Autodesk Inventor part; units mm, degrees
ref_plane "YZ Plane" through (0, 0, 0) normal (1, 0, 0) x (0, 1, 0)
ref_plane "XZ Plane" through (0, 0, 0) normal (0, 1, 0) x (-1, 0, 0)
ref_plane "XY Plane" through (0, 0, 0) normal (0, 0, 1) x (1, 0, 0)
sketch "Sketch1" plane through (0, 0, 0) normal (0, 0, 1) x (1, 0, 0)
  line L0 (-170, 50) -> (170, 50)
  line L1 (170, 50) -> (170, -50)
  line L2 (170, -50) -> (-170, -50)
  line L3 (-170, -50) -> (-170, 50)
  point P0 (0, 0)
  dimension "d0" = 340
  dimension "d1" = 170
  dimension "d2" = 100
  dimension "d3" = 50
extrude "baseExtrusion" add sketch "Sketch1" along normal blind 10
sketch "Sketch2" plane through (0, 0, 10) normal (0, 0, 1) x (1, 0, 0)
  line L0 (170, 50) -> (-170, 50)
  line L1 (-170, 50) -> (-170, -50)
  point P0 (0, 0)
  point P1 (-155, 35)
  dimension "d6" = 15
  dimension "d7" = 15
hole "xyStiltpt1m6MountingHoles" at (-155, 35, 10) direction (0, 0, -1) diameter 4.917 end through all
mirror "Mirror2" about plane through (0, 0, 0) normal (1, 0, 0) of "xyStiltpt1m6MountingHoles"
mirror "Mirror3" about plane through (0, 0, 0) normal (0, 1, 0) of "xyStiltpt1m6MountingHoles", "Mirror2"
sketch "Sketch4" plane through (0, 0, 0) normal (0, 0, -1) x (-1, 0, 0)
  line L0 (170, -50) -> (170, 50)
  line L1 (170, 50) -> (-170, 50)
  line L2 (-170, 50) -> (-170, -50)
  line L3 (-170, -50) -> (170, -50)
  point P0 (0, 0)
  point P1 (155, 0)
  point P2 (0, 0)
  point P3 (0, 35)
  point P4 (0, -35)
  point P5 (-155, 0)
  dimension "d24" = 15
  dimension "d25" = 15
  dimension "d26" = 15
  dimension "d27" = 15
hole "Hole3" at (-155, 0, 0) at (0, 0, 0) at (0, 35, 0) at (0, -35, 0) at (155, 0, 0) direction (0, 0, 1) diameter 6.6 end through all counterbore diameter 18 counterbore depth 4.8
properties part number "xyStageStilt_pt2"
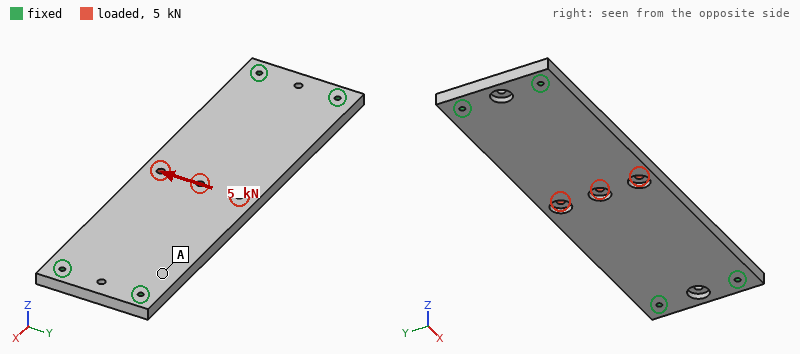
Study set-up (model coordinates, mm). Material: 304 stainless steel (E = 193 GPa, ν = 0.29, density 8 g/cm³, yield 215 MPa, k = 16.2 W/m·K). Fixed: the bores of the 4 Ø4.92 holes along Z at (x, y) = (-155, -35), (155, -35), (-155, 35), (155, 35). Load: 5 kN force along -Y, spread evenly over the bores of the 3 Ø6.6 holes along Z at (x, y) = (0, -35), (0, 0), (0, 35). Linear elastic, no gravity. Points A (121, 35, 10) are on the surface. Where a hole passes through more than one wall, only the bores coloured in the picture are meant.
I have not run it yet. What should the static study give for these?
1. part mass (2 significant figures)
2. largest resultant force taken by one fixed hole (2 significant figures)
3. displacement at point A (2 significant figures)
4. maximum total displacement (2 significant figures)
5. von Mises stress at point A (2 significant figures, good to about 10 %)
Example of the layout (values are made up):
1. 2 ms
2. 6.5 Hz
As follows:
1. 2.7 kg
2. 2.9 kN
3. 3.5 µm
4. 21 µm
5. 6.7 MPa
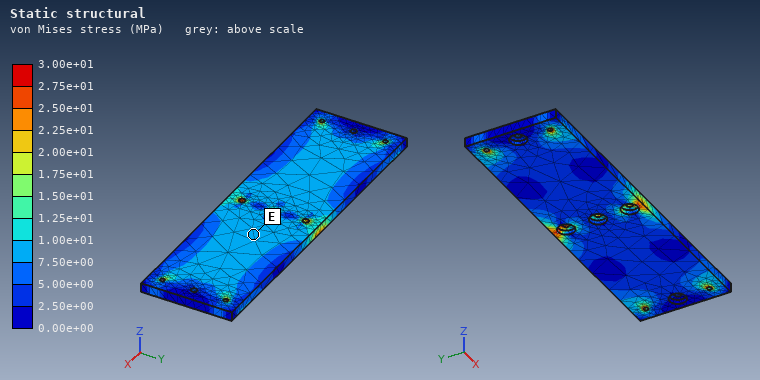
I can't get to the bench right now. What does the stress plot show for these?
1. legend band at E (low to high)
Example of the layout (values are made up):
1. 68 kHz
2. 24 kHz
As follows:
1. 7.50e+00 to 1.00e+01 MPa
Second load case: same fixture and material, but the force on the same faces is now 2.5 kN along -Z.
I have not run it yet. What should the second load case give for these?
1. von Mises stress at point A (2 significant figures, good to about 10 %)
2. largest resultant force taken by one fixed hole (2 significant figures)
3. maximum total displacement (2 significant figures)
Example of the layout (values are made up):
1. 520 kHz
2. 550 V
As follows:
1. 30 MPa
2. 720 N
3. 0.31 mm
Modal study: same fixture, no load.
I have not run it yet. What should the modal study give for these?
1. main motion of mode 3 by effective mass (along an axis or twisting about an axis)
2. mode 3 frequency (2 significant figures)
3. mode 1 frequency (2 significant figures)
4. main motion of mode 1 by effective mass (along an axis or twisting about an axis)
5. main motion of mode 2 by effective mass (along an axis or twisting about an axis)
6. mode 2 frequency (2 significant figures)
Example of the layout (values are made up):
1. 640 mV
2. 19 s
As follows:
1. twisting about Y
2. 1300 Hz
3. 470 Hz
4. along Z
5. twisting about X
6. 1100 Hz
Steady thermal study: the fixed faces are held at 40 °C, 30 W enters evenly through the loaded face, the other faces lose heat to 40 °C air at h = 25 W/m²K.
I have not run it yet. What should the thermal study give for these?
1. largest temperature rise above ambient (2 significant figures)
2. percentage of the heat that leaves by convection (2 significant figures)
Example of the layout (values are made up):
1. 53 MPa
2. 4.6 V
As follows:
1. 66 K
2. 91 %
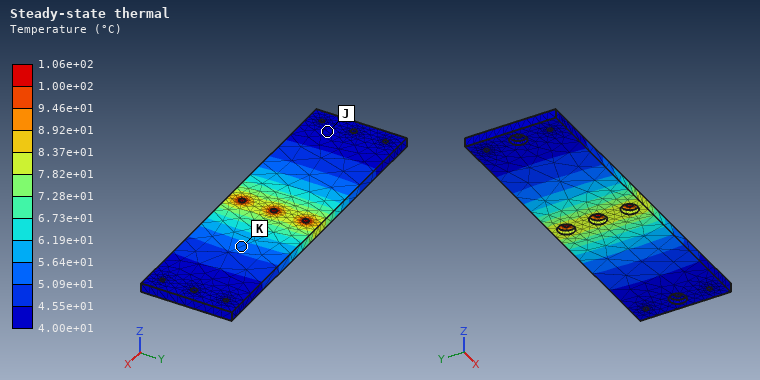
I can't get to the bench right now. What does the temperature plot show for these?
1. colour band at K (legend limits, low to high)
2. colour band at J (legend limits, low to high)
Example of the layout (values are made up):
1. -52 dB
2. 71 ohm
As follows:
1. 5.09e+01 to 5.64e+01 °C
2. 4.00e+01 to 4.55e+01 °C
